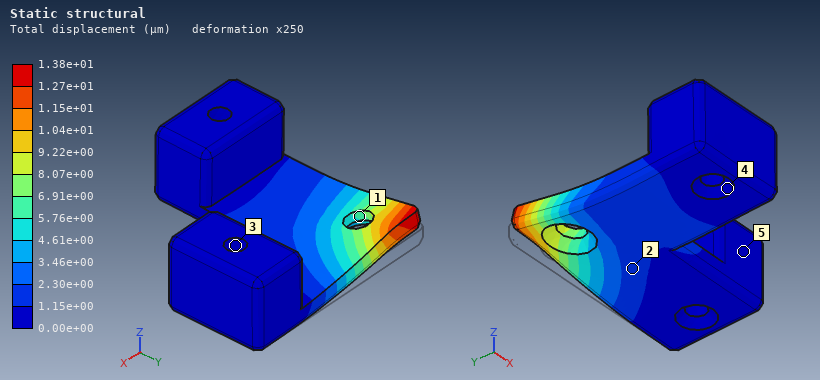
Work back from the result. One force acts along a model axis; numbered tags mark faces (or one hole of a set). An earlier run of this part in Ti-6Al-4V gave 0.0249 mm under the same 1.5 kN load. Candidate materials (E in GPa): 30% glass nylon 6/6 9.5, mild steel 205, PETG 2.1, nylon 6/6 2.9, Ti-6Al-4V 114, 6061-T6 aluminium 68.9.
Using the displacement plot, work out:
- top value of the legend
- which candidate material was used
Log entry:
1.38e+01 µm
mild steel
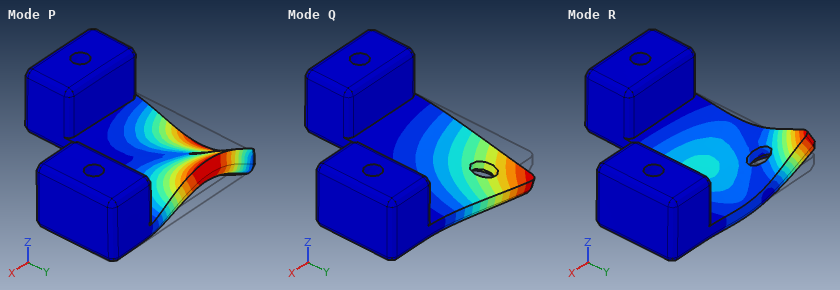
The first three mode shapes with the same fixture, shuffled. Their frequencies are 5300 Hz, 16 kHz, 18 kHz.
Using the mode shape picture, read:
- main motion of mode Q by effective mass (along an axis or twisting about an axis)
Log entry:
along Z
